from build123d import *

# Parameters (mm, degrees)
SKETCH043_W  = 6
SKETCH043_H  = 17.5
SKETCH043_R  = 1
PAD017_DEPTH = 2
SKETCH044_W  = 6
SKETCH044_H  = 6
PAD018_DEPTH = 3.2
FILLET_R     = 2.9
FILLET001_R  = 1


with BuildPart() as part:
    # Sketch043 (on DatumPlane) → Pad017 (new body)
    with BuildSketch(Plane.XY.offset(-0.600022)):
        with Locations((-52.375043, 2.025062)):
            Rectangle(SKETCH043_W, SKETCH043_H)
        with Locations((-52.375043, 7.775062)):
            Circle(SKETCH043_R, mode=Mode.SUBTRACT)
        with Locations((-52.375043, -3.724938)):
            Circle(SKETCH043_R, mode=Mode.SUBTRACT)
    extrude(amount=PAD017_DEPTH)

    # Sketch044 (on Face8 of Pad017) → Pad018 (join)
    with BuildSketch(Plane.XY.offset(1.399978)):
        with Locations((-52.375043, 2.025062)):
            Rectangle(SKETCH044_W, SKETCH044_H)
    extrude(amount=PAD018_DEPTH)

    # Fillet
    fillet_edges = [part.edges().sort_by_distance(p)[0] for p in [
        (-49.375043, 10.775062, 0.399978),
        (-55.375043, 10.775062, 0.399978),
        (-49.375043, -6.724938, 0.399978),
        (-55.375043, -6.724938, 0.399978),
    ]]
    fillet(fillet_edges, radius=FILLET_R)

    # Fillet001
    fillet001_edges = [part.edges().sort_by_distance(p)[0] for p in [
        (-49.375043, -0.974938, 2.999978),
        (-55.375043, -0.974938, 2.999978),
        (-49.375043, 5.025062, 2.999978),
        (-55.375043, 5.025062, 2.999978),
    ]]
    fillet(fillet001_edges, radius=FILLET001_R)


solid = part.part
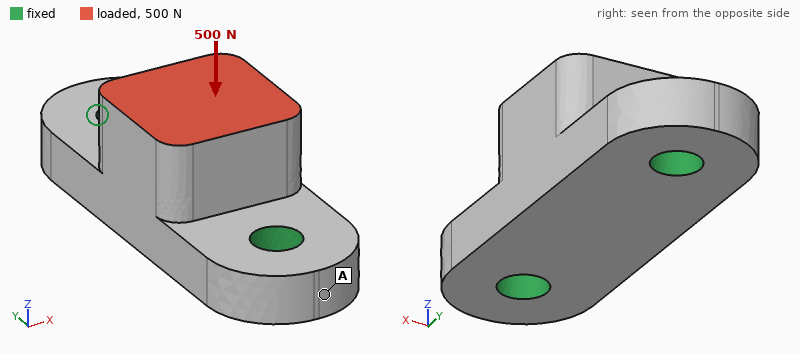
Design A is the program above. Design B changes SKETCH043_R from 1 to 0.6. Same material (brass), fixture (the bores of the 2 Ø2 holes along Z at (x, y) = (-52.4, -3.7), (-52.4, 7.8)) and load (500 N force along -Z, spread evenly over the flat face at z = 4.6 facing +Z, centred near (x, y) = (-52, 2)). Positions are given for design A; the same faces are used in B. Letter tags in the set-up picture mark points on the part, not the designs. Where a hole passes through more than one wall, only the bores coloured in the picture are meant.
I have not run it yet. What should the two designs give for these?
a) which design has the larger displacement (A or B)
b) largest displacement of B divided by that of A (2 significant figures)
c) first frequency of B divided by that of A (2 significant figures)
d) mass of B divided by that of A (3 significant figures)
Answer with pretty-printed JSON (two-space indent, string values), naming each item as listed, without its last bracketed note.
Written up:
{
  "which design has the larger displacement": "B",
  "largest displacement of B divided by that of A": "1.4",
  "first frequency of B divided by that of A": "0.86",
  "mass of B divided by that of A": "1.03"
}
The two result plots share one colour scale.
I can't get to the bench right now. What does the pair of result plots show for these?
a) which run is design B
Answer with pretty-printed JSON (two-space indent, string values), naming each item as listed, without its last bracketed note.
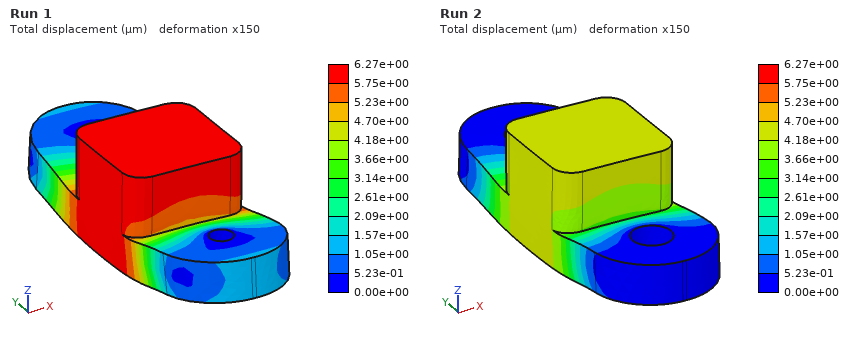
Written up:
{
  "which run is design B": "Run 1"
}
